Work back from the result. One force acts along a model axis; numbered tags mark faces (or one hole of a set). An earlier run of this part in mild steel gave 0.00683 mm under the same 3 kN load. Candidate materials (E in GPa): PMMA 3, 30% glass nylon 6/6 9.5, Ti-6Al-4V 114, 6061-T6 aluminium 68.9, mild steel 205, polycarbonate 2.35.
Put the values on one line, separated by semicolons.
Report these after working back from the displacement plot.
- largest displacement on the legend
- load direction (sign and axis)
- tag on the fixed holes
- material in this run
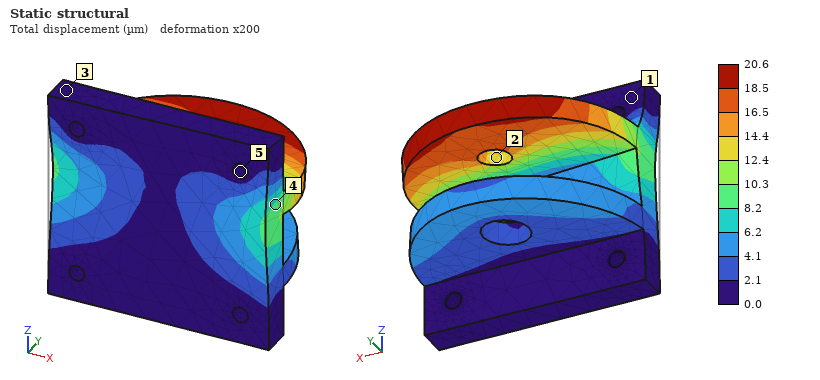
20.6 µm; +X; 5; 6061-T6 aluminium
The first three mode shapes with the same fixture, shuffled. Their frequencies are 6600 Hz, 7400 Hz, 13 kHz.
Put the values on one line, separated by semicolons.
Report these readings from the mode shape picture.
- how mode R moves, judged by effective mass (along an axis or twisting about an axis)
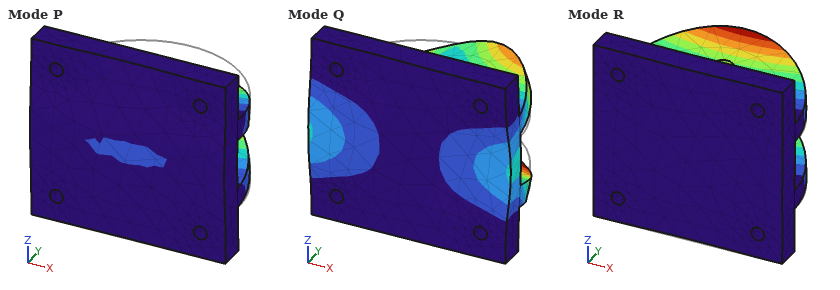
along Z
